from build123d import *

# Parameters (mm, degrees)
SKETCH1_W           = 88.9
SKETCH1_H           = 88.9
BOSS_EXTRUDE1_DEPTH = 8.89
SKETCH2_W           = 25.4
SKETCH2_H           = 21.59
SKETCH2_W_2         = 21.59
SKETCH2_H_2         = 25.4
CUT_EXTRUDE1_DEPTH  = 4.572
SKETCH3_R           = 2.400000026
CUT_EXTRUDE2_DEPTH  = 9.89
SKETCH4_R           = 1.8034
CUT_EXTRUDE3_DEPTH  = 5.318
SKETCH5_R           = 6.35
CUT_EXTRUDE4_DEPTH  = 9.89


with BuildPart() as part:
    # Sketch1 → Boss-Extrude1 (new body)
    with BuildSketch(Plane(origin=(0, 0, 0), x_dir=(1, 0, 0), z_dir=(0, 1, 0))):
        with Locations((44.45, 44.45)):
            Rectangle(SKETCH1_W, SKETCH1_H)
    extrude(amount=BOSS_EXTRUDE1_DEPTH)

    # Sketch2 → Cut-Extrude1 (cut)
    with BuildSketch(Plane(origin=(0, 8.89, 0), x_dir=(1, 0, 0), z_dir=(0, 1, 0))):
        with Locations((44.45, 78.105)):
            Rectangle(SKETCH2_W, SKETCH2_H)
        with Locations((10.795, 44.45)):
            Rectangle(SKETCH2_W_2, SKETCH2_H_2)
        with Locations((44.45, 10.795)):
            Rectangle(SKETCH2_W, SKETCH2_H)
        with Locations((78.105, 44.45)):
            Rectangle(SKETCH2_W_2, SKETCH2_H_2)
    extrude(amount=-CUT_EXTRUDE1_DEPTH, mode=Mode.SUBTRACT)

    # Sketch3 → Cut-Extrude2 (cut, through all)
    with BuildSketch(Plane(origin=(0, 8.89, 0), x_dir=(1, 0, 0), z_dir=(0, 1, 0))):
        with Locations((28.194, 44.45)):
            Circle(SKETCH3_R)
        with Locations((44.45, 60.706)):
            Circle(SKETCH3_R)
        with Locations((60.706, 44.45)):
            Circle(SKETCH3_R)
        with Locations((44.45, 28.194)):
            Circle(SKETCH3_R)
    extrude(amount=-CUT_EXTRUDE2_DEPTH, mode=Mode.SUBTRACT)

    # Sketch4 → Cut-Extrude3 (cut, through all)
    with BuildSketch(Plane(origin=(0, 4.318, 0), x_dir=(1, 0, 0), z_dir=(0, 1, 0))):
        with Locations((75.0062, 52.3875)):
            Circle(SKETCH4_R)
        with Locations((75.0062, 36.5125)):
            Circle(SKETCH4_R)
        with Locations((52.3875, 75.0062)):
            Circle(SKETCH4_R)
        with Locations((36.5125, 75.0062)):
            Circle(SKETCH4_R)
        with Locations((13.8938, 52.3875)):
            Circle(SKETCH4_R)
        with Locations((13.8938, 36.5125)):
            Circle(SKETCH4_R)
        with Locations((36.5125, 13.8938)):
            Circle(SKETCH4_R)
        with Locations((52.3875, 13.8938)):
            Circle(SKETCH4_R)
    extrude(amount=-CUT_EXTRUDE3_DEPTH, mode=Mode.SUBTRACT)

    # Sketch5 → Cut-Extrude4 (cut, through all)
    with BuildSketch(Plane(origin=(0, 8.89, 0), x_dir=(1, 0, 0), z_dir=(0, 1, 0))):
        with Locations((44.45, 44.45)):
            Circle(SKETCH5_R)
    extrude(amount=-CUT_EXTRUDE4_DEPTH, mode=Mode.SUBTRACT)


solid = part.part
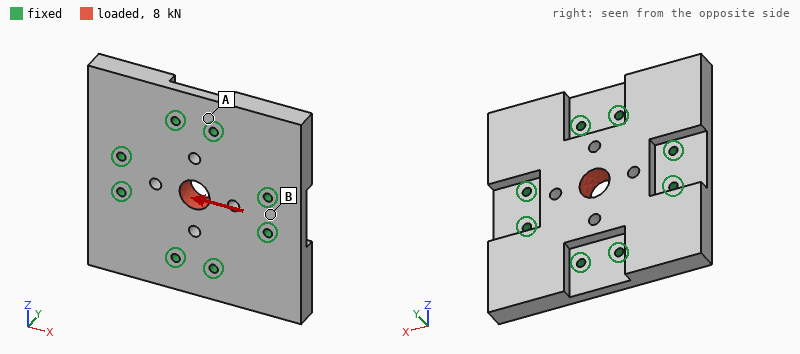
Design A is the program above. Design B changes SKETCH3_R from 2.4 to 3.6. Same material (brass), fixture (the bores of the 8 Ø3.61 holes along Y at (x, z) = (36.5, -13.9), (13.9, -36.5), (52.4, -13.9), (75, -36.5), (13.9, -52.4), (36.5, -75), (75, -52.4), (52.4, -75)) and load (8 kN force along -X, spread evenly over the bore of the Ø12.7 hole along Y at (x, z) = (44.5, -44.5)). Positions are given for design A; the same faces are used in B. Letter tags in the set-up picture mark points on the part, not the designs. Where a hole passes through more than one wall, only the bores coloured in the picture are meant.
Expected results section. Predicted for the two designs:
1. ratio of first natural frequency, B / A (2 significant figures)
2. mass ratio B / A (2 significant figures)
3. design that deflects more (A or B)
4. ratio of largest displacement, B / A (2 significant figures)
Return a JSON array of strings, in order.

["0.99", "0.99", "B", "1.1"]
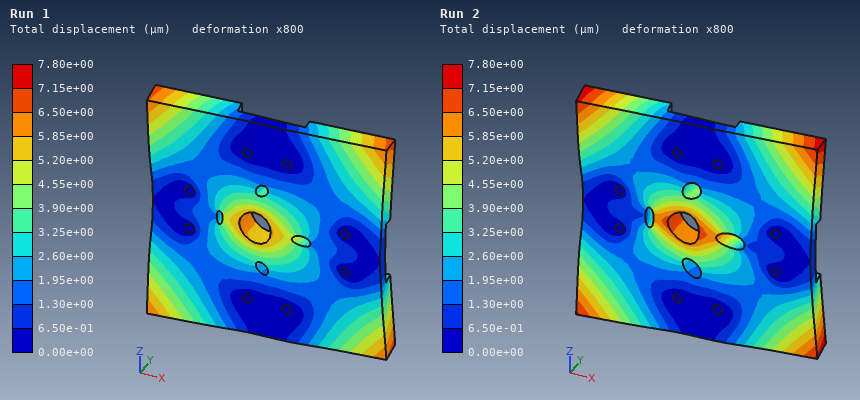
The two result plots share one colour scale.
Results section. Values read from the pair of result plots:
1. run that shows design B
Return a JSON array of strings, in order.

["Run 2"]
